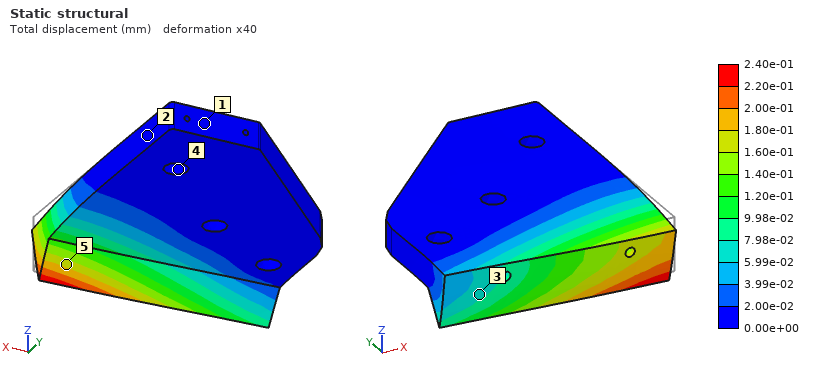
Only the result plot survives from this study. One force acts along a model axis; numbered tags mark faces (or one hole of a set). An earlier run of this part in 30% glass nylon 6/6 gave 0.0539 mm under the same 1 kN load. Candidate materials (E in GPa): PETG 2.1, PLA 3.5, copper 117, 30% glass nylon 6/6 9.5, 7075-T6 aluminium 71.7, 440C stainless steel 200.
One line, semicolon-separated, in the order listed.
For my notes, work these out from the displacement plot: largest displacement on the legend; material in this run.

2.40e-01 mm; PETG
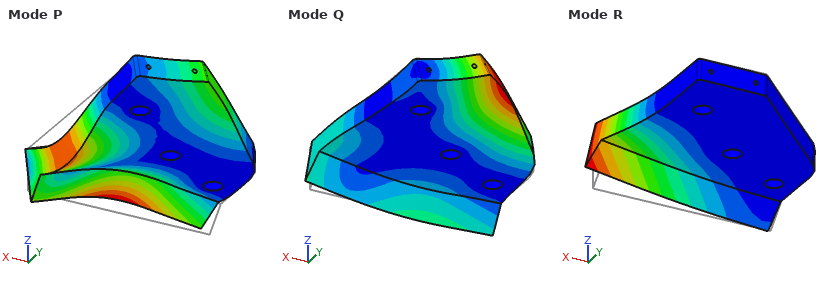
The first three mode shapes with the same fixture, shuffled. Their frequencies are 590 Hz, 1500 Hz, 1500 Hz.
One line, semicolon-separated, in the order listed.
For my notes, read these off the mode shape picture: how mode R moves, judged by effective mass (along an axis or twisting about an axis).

along Z
